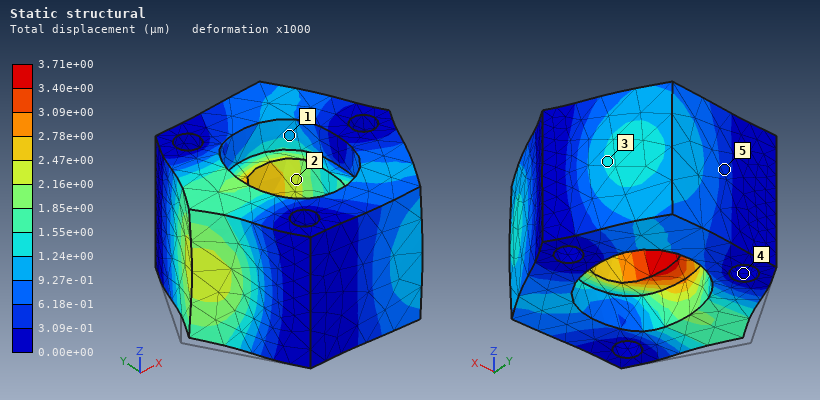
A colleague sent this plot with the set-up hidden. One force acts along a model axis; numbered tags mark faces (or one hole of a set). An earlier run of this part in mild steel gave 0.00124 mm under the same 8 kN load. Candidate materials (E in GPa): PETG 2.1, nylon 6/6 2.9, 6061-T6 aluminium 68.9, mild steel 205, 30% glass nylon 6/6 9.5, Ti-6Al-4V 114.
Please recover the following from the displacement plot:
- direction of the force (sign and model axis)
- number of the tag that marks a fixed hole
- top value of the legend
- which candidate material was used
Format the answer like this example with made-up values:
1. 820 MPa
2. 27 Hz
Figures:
1. +X
2. 4
3. 3.71e+00 µm
4. 6061-T6 aluminium
